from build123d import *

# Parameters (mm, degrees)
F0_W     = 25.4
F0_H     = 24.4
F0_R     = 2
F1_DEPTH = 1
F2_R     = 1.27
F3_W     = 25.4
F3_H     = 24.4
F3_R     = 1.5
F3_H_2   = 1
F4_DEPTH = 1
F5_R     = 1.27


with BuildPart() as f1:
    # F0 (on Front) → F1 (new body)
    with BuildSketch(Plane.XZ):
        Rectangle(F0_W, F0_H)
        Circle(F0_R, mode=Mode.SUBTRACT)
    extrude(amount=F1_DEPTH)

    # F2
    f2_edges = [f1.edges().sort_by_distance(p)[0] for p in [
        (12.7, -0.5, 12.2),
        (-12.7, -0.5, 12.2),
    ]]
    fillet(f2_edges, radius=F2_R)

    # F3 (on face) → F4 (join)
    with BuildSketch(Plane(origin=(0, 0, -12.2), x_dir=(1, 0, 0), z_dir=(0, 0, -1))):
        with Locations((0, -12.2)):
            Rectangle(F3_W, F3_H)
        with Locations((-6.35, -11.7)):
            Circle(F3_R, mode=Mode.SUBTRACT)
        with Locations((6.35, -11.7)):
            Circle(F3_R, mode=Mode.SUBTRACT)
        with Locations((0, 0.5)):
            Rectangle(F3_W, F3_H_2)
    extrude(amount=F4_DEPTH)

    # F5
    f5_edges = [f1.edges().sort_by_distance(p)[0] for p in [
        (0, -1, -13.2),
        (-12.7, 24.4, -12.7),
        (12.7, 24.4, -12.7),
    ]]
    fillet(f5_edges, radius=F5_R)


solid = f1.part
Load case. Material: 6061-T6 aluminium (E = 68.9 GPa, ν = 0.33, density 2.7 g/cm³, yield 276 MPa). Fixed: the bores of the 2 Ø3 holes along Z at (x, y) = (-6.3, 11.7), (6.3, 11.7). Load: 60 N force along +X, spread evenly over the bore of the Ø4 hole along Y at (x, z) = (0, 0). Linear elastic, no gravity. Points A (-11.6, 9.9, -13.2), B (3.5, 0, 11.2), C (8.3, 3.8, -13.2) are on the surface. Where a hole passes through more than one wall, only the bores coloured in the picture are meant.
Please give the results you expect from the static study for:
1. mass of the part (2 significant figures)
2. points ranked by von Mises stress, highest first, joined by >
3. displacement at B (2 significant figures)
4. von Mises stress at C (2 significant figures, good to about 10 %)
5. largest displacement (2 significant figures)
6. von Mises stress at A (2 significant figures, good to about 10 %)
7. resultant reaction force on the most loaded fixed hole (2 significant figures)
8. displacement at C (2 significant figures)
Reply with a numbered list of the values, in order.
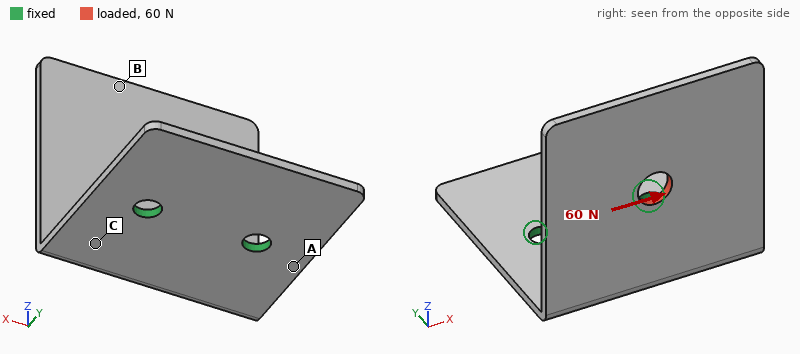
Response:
1. 3.3 g
2. A > C > B
3. 0.40 mm
4. 60 MPa
5. 0.47 mm
6. 95 MPa
7. 73 N
8. 0.076 mm
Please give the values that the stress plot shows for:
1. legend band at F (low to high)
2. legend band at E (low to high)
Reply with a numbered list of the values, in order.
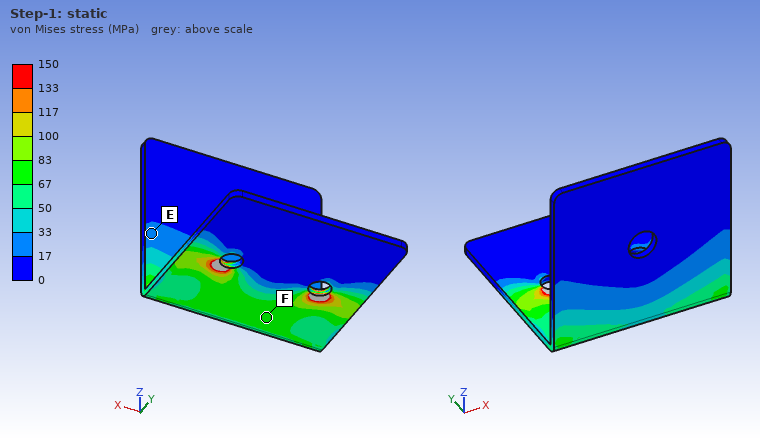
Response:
1. 67 to 83 MPa
2. 17 to 33 MPa
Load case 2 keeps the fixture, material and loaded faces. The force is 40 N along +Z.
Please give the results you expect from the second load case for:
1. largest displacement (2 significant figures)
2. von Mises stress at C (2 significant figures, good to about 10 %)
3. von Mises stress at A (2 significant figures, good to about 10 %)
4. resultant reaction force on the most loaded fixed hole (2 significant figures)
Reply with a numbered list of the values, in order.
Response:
1. 0.45 mm
2. 36 MPa
3. 58 MPa
4. 20 N
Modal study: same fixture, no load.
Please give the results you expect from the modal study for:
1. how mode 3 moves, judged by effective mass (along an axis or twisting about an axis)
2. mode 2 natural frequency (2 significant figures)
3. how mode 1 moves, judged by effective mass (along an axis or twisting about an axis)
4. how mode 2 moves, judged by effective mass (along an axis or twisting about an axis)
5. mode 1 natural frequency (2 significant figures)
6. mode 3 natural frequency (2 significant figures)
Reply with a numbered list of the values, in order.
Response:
1. along Z
2. 1600 Hz
3. along Y
4. along X
5. 780 Hz
6. 2800 Hz
